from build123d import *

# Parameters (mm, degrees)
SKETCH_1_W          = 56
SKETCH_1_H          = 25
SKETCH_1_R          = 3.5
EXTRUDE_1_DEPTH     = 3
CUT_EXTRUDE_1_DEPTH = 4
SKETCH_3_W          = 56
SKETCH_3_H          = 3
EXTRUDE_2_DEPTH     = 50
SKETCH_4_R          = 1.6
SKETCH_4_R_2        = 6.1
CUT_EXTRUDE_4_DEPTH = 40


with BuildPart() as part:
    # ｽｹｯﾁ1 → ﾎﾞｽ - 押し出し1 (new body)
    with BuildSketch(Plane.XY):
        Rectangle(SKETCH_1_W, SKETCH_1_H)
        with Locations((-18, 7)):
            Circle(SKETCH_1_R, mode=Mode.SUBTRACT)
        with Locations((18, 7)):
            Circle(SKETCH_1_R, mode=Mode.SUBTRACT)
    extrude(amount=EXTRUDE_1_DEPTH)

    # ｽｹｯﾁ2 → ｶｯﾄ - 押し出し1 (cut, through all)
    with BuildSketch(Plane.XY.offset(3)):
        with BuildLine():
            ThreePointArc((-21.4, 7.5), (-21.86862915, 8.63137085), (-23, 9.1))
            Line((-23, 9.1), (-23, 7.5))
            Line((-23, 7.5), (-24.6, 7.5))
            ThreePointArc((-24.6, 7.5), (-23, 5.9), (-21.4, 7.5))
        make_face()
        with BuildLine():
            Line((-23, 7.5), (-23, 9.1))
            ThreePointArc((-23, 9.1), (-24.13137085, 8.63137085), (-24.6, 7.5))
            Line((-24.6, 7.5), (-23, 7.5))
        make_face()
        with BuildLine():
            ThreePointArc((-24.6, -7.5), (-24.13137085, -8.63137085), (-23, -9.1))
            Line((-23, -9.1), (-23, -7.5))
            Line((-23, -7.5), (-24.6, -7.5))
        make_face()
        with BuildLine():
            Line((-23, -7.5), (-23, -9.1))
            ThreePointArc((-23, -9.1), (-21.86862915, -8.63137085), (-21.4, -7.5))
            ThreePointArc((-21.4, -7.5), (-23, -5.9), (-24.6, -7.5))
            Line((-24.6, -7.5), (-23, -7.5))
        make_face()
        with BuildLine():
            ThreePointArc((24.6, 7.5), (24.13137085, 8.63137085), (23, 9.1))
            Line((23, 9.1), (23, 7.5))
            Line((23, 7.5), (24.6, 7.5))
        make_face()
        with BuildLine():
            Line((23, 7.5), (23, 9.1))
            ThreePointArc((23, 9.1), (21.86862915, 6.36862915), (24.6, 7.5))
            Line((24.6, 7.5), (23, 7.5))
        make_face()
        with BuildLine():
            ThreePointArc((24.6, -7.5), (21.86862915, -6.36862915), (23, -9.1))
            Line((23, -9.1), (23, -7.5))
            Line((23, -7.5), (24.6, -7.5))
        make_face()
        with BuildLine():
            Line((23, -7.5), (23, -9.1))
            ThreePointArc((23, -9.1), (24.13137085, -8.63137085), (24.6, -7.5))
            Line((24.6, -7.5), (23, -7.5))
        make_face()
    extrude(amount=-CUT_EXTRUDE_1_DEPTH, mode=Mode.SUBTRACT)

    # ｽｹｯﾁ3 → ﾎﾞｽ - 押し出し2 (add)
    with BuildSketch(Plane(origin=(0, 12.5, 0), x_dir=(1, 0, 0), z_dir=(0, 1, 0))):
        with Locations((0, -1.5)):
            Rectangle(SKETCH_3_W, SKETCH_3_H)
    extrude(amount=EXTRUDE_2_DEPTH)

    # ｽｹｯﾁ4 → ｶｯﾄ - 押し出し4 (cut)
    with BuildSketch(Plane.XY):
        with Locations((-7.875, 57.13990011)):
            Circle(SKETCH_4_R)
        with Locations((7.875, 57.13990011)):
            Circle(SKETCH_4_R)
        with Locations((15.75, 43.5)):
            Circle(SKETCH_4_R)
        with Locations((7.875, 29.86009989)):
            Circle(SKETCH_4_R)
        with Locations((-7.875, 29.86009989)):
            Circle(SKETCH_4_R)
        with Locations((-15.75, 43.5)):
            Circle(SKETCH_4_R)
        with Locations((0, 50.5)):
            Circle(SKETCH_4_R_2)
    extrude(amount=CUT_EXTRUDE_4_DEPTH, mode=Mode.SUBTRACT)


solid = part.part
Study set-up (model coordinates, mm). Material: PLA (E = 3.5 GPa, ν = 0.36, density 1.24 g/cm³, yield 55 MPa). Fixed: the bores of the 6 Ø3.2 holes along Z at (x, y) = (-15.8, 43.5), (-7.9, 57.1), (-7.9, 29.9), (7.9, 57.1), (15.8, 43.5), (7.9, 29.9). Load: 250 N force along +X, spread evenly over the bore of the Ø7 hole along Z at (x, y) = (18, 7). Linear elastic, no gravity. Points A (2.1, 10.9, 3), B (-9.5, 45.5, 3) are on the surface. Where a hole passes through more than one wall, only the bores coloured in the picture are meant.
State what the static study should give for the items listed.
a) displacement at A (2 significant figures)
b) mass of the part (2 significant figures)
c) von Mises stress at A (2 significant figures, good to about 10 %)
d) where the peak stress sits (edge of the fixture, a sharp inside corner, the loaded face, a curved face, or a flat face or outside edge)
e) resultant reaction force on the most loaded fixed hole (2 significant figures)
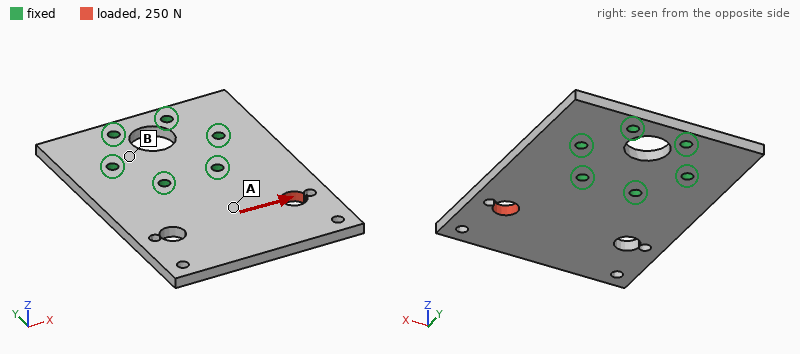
0.045 mm
15 g
3.6 MPa
the loaded face
170 N
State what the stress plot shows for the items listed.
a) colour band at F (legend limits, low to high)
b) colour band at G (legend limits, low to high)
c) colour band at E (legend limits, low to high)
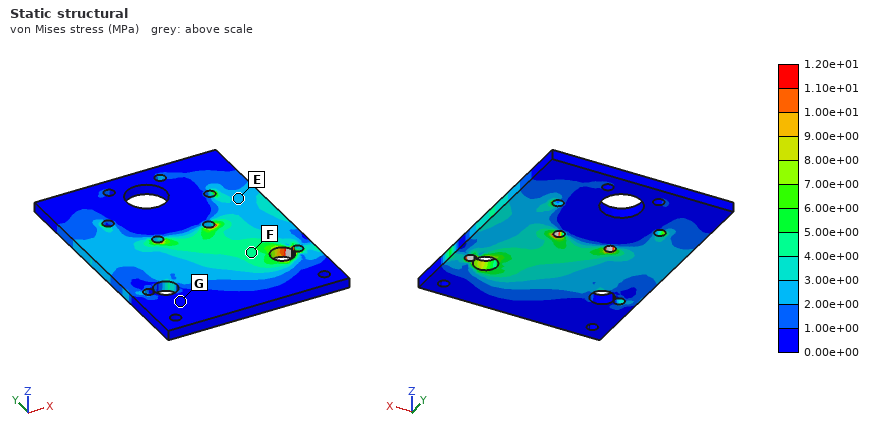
4.00e+00 to 5.00e+00 MPa
0.00e+00 to 1.00e+00 MPa
2.00e+00 to 3.00e+00 MPa
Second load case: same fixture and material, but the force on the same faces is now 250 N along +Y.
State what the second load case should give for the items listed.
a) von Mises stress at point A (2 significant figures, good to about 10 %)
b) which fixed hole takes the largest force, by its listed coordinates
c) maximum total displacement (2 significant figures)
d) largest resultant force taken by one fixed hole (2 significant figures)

1.2 MPa
(7.9, 29.9)
76 µm
150 N
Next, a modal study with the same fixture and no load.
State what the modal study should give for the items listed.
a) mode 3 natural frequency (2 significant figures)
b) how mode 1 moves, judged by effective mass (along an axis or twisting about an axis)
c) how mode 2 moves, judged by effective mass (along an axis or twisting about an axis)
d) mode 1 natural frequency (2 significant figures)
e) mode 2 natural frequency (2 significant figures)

1800 Hz
along Z
twisting about Y
440 Hz
770 Hz
